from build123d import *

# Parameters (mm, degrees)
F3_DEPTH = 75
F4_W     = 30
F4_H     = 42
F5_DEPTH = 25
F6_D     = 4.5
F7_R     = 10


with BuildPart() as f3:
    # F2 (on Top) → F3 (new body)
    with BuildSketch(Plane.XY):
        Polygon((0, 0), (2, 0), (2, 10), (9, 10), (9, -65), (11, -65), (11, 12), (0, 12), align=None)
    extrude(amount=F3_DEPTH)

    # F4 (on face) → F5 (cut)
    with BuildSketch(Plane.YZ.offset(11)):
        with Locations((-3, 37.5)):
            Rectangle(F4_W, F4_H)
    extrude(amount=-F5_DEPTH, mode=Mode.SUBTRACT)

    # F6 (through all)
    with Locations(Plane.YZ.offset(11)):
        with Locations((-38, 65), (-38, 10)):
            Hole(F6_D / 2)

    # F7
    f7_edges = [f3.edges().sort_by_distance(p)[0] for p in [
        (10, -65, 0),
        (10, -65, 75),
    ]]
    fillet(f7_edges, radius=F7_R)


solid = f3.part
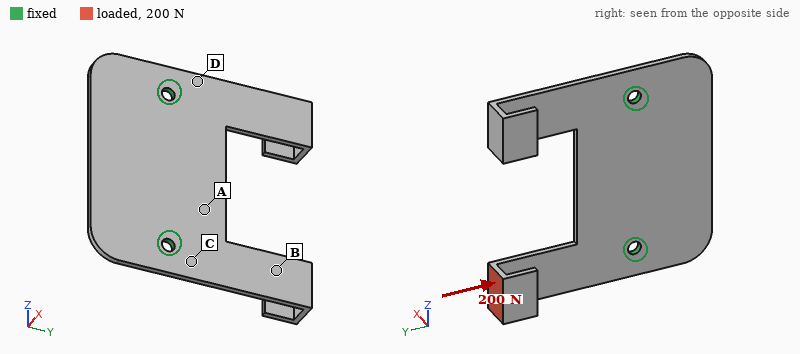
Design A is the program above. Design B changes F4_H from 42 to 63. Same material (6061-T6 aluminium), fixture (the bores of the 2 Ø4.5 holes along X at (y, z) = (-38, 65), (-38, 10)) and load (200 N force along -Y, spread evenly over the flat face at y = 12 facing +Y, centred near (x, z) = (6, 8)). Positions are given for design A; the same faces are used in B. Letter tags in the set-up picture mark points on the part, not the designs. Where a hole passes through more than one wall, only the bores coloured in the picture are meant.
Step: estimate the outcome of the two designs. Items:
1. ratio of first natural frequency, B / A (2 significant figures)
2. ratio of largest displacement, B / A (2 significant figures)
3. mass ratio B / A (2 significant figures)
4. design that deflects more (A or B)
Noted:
1.2
2.2
0.80
B
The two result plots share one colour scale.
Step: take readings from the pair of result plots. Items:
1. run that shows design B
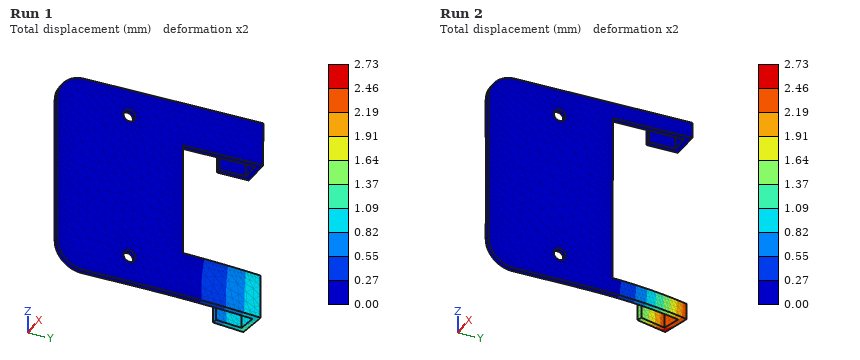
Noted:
Run 2
